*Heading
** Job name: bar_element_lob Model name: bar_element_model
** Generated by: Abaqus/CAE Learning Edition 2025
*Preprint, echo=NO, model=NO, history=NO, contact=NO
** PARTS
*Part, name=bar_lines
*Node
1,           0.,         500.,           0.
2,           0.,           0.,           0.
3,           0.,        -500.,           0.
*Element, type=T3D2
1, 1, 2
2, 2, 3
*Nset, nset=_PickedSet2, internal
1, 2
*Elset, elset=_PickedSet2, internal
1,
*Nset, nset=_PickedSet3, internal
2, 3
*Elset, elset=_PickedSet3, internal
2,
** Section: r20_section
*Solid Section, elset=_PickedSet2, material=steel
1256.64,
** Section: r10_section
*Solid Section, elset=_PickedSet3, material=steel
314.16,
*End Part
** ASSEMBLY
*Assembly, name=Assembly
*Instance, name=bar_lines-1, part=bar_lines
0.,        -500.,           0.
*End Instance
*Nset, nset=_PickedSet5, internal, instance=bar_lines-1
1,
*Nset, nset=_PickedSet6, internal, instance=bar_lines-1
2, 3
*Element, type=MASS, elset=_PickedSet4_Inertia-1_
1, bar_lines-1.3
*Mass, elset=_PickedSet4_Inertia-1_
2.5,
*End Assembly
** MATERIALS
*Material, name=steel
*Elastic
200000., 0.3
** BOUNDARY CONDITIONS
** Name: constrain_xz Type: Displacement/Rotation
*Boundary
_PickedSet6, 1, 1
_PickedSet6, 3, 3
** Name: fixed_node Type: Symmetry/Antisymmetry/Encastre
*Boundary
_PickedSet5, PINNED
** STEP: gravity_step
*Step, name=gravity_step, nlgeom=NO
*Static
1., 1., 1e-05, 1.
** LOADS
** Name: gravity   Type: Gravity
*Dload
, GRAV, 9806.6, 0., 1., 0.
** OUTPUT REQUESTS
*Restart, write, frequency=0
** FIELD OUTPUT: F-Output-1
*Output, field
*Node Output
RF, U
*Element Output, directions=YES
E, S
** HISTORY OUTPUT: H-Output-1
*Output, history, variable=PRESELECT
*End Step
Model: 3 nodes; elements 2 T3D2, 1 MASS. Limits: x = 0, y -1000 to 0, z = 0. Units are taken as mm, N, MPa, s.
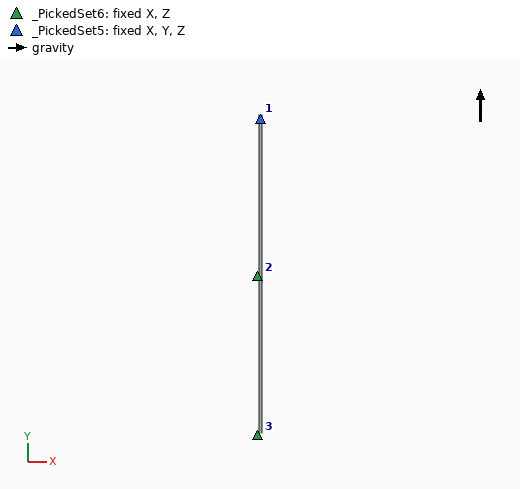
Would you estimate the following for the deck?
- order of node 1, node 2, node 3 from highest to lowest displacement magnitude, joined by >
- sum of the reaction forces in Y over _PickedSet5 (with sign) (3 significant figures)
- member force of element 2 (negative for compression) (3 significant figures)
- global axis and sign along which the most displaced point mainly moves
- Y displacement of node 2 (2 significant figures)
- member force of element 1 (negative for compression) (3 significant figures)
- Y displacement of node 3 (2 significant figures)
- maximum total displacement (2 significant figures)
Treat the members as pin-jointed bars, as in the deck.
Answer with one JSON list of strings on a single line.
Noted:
["node 3 > node 2 > node 1", "-24500 N", "-24500 N", "+Y", "0.049 mm", "-24500 N", "0.24 mm", "0.24 mm"]
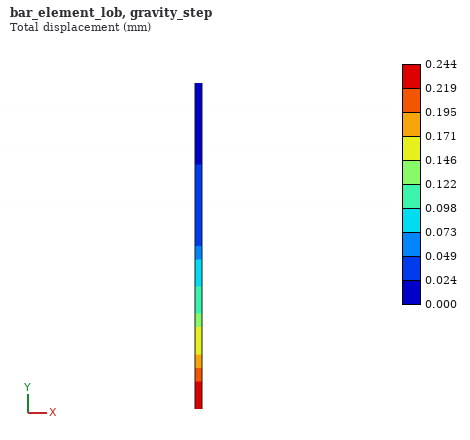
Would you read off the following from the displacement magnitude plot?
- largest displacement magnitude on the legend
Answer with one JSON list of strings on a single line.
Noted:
["0.244 mm"]
